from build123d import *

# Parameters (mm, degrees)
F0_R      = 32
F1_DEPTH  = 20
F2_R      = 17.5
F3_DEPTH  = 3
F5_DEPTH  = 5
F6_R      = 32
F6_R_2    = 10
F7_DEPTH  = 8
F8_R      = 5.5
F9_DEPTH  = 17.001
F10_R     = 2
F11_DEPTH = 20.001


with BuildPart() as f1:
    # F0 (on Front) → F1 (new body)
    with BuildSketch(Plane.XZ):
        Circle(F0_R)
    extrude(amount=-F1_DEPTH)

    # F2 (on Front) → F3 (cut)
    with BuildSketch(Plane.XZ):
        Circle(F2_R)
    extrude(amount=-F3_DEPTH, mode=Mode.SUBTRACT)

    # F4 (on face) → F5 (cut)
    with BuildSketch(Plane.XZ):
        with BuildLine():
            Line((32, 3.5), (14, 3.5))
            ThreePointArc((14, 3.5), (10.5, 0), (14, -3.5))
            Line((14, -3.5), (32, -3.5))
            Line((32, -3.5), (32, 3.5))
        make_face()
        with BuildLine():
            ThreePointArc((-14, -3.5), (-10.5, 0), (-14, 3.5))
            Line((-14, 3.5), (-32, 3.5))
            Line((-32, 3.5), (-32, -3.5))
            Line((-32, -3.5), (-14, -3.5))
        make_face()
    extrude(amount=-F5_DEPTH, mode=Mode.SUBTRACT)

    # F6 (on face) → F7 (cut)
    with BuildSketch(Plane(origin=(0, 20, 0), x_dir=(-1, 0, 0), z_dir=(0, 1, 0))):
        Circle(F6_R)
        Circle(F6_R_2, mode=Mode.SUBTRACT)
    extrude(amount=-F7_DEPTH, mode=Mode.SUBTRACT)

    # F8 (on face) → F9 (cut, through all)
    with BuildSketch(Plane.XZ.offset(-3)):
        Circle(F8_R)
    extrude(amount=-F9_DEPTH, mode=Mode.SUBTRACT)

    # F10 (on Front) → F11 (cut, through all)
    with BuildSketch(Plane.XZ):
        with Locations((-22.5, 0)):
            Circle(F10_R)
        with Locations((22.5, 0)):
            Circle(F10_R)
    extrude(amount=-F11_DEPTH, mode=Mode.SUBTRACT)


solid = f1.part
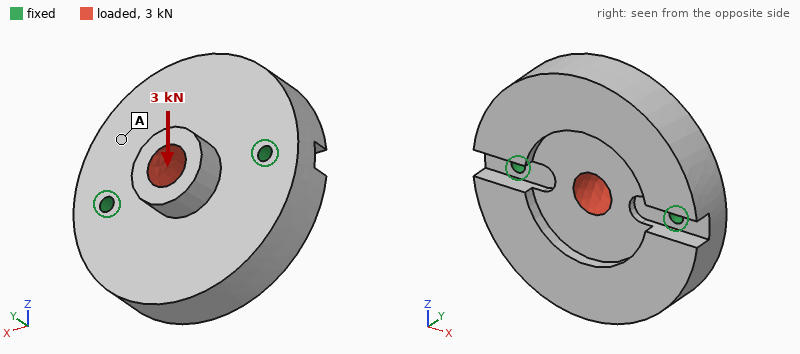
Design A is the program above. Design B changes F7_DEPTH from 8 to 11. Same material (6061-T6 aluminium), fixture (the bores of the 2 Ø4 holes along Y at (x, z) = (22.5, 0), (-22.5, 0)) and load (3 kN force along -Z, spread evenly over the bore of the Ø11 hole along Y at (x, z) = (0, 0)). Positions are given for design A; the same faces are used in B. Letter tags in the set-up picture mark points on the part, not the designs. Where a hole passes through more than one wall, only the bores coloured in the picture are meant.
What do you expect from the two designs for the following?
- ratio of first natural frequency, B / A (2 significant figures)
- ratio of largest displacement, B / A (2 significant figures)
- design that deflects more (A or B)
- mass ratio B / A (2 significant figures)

0.63
4.6
B
0.76
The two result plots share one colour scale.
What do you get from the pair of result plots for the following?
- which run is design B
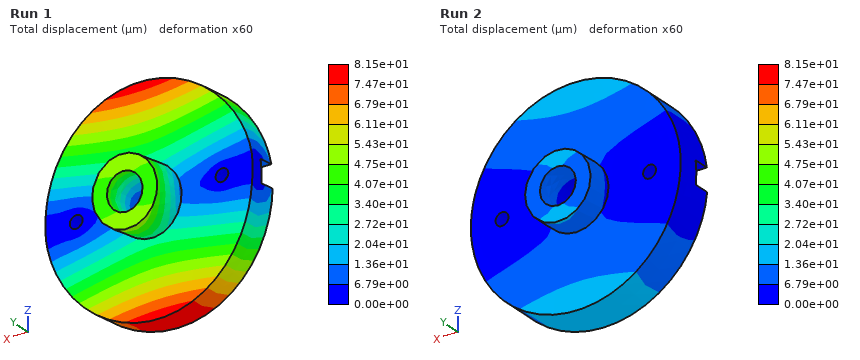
Run 1
